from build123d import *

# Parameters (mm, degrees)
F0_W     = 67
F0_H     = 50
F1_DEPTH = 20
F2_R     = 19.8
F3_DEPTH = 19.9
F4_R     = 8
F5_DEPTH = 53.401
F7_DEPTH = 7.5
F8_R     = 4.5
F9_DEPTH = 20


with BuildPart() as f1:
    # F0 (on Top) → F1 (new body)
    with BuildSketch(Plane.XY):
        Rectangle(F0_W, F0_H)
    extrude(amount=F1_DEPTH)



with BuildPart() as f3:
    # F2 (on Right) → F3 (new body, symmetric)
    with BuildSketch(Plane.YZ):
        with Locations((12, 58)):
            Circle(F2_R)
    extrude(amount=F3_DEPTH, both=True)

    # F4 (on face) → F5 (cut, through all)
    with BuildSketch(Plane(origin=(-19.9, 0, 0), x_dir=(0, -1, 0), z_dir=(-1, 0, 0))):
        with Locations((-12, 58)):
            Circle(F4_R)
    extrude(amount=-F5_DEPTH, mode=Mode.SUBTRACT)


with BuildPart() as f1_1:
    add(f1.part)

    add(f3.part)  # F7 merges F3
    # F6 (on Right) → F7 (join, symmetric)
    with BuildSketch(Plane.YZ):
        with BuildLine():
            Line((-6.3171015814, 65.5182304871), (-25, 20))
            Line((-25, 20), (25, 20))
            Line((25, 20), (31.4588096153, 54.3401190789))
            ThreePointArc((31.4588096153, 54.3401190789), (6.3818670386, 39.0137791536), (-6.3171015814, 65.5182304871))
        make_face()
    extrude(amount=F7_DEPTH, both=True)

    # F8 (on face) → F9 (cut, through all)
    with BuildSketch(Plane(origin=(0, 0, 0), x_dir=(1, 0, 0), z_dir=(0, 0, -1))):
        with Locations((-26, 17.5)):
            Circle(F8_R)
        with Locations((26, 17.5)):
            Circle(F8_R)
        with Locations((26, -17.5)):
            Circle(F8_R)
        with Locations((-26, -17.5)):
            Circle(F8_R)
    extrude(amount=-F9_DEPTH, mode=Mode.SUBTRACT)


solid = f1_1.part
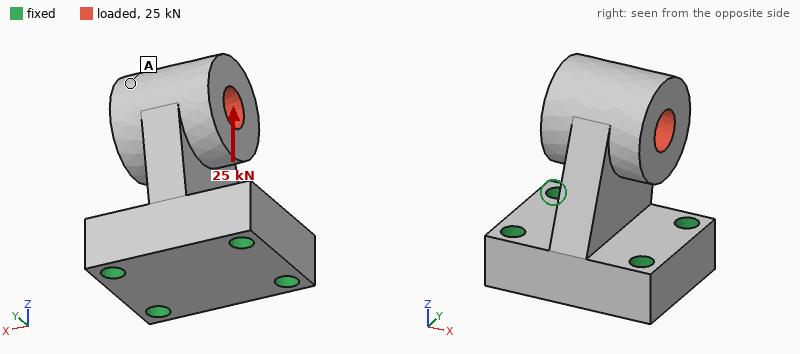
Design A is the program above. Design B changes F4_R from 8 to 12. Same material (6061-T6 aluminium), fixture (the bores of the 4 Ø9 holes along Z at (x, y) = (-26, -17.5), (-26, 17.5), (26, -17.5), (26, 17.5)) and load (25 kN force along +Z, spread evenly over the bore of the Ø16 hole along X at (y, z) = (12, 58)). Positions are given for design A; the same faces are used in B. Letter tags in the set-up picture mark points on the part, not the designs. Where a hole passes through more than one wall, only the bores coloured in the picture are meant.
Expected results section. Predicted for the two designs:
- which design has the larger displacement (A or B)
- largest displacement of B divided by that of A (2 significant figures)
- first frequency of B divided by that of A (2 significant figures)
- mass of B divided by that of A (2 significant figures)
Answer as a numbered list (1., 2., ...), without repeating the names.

1. B
2. 1.2
3. 1.1
4. 0.92
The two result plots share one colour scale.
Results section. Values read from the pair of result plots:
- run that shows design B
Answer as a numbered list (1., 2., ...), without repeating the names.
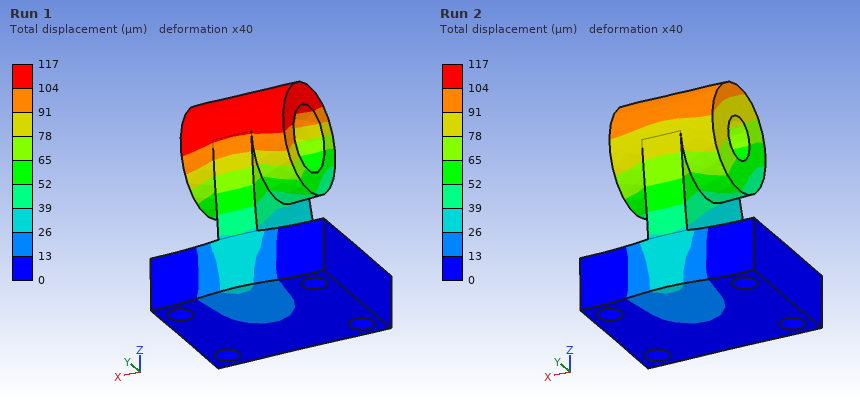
1. Run 1
